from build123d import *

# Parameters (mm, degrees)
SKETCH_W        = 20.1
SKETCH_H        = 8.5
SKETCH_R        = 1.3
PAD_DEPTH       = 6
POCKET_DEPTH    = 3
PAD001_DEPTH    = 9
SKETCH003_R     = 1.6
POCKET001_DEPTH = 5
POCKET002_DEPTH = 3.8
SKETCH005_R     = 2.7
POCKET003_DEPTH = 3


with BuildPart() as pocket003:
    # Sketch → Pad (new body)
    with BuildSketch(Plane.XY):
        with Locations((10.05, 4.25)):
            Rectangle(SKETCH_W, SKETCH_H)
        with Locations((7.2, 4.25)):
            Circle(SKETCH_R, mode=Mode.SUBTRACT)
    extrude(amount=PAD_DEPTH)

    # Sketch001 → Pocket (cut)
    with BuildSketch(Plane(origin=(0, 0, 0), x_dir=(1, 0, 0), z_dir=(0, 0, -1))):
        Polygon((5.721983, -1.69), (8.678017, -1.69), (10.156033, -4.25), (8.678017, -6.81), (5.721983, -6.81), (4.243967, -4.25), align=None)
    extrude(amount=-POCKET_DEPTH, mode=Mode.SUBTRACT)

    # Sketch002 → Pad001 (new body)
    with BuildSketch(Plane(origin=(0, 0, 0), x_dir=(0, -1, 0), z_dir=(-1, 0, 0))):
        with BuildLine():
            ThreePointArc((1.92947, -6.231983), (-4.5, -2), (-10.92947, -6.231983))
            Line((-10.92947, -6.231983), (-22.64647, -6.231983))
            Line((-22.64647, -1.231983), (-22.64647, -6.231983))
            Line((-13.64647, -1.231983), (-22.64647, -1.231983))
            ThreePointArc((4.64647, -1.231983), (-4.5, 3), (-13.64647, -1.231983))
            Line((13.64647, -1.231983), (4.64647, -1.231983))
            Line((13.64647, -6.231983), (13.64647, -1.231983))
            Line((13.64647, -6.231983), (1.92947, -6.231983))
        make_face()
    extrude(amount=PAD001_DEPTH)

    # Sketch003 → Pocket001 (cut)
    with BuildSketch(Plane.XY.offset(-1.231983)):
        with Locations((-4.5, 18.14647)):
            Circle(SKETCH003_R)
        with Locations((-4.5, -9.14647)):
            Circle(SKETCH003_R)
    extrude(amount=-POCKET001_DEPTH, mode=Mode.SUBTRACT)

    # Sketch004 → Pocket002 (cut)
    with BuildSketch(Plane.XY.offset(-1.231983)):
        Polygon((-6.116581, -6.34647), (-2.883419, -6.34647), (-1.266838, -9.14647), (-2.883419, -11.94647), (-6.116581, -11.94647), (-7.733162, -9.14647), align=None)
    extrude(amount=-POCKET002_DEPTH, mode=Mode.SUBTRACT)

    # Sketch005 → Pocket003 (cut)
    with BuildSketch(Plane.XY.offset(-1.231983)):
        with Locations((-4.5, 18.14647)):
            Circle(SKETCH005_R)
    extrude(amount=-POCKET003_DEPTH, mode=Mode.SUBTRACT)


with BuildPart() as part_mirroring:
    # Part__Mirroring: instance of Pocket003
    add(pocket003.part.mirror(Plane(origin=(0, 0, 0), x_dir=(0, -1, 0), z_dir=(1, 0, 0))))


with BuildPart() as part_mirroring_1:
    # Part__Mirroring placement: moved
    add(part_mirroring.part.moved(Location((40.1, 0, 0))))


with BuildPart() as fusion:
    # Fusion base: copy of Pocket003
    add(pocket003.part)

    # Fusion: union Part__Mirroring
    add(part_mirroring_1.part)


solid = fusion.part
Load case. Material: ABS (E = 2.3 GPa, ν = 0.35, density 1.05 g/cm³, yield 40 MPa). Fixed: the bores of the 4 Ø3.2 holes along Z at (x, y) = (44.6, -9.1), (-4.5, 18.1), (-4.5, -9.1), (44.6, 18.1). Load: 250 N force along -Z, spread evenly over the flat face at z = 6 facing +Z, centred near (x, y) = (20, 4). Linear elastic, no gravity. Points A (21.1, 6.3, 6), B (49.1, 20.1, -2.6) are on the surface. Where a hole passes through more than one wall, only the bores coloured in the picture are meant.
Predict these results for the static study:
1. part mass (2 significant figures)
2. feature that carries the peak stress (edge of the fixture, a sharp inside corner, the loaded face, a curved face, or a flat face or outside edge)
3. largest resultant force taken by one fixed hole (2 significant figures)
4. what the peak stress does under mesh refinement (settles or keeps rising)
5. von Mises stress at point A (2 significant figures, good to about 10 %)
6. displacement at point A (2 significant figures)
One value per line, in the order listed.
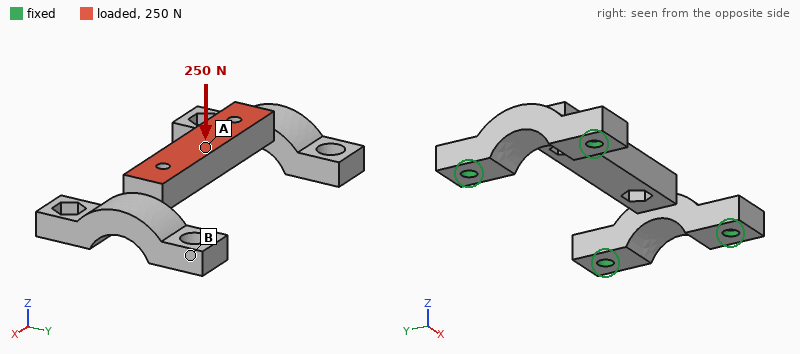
5.3 g
edge of the fixture
120 N
keeps rising
17 MPa
0.48 mm
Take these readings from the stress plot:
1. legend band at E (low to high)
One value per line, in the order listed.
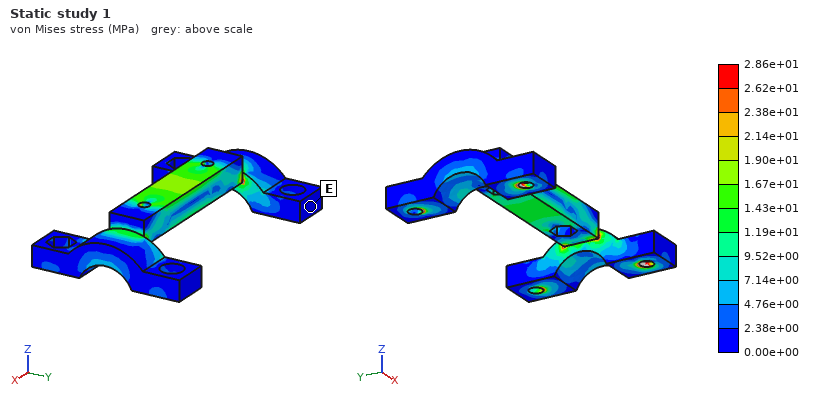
0.00e+00 to 2.38e+00 MPa
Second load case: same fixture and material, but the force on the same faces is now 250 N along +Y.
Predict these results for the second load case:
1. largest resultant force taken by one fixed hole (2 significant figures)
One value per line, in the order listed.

100 N
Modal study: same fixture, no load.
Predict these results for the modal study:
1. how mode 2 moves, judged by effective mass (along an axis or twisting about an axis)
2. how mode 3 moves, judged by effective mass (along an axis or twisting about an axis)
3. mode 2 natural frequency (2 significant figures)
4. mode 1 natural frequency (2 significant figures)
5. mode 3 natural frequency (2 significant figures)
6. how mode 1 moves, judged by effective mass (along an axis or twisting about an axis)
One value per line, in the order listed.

along X
along Y
2900 Hz
2800 Hz
3700 Hz
along Z
